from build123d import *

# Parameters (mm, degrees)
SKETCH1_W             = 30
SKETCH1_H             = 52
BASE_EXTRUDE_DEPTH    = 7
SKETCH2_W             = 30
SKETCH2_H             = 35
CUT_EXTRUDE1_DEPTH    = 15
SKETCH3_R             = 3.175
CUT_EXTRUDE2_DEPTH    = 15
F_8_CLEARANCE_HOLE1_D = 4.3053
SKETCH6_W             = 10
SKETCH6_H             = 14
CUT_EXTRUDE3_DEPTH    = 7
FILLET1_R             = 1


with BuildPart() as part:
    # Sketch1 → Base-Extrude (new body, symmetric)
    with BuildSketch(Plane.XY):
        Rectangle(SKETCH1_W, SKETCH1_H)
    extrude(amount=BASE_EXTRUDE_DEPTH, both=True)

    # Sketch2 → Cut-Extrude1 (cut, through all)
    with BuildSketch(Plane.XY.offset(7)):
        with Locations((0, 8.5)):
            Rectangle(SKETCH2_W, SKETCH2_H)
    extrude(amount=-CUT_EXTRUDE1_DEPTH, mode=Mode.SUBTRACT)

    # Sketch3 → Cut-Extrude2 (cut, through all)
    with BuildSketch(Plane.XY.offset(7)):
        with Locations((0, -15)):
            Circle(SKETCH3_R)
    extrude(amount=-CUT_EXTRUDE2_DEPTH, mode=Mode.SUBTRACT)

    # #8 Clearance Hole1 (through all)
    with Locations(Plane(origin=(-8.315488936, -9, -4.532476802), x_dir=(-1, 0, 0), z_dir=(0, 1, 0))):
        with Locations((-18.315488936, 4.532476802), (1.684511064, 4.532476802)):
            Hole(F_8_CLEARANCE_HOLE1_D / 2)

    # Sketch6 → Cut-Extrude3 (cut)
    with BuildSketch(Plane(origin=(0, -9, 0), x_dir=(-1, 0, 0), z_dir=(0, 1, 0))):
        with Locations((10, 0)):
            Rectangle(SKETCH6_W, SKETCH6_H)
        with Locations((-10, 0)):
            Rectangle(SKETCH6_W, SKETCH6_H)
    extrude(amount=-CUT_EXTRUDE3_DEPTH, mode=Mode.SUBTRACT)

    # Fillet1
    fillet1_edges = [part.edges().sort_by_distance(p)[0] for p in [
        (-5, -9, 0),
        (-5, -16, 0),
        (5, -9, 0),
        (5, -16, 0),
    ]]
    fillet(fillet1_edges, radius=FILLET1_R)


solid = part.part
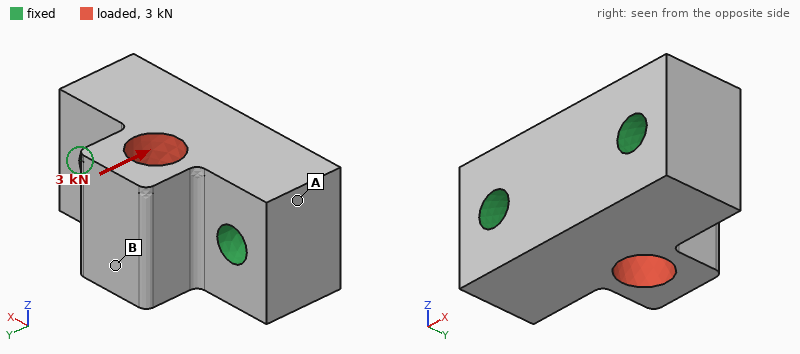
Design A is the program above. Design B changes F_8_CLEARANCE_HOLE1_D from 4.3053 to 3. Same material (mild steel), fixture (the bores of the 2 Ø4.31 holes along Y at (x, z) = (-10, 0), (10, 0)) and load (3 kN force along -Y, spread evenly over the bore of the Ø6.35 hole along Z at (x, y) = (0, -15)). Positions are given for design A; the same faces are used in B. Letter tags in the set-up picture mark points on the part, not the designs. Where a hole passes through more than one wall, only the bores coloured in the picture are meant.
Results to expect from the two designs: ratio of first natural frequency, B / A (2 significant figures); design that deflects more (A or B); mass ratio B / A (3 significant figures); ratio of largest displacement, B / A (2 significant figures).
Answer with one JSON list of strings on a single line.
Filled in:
["0.92", "B", "1.03", "1.1"]
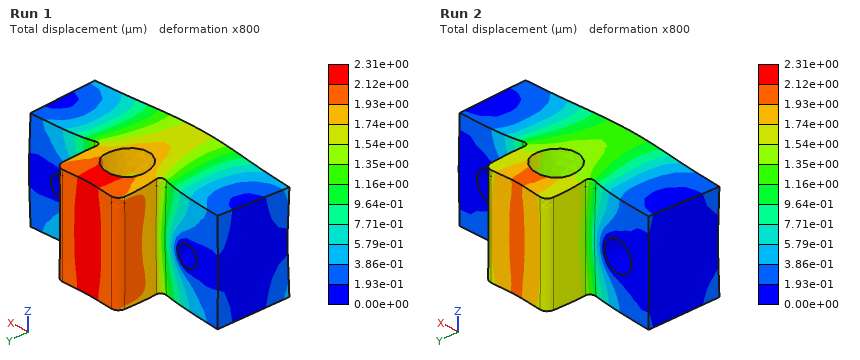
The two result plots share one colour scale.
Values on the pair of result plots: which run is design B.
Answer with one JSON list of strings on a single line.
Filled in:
["Run 1"]
